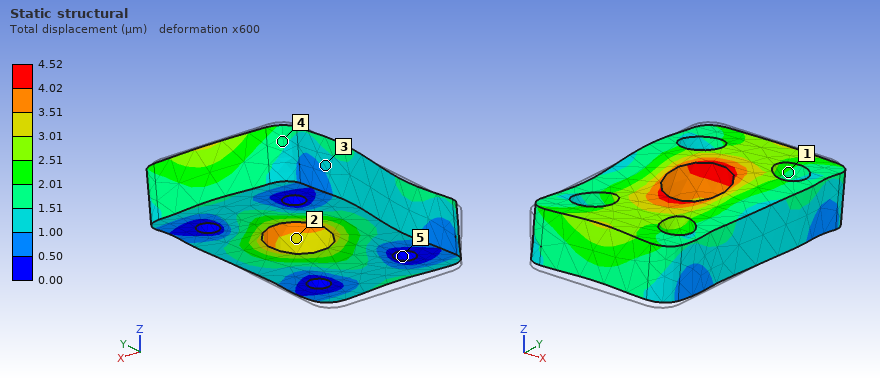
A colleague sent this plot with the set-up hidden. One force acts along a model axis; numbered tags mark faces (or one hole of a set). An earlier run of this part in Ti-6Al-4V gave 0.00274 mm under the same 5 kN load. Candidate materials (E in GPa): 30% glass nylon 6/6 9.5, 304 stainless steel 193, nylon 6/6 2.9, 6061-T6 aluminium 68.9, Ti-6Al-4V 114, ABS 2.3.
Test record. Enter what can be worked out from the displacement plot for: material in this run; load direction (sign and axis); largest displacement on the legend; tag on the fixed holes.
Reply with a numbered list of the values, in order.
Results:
1. 6061-T6 aluminium
2. +Y
3. 4.52 µm
4. 5
